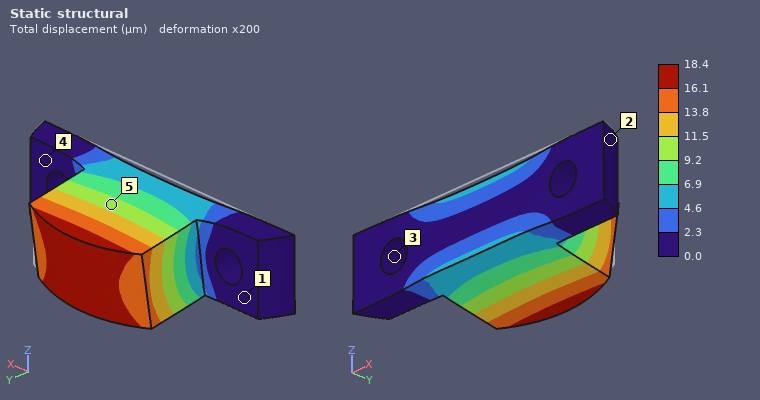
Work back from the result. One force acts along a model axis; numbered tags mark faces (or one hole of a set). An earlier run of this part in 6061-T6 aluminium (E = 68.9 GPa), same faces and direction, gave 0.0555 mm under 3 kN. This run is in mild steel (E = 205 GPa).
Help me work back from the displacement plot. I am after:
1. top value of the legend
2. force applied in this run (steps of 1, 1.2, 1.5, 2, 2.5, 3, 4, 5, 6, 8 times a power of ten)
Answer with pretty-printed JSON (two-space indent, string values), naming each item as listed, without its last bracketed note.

{
  "top value of the legend": "18.4 µm",
  "force applied in this run": "3 kN"
}
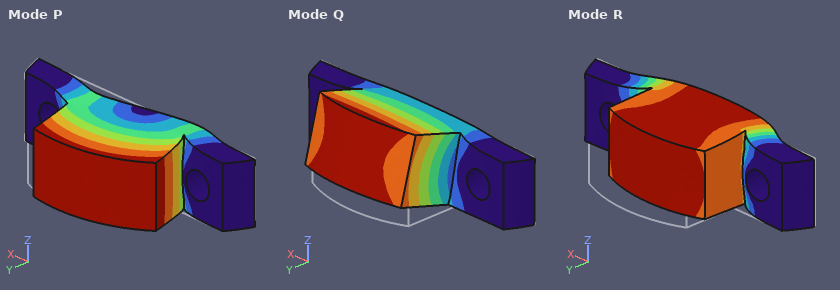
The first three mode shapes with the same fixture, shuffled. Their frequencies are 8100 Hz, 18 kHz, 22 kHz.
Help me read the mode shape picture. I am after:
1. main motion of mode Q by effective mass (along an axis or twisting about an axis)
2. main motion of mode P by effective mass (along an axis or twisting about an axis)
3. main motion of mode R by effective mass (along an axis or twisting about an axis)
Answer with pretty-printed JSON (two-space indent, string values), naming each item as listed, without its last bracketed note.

{
  "main motion of mode Q by effective mass": "along Z",
  "main motion of mode P by effective mass": "along X",
  "main motion of mode R by effective mass": "along Y"
}
